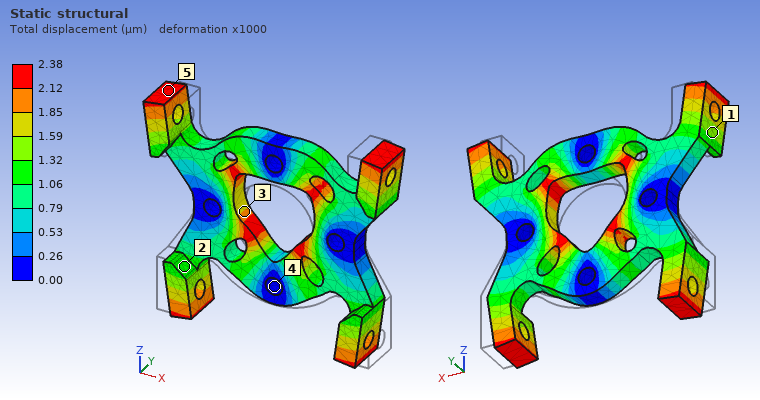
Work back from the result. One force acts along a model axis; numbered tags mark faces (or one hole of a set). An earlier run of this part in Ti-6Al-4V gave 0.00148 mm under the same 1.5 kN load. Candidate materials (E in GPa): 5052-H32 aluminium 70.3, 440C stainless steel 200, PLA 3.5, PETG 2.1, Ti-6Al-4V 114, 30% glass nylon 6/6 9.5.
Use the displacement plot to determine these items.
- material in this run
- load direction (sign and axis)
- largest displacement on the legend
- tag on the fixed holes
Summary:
5052-H32 aluminium
+Z
2.38 µm
4
